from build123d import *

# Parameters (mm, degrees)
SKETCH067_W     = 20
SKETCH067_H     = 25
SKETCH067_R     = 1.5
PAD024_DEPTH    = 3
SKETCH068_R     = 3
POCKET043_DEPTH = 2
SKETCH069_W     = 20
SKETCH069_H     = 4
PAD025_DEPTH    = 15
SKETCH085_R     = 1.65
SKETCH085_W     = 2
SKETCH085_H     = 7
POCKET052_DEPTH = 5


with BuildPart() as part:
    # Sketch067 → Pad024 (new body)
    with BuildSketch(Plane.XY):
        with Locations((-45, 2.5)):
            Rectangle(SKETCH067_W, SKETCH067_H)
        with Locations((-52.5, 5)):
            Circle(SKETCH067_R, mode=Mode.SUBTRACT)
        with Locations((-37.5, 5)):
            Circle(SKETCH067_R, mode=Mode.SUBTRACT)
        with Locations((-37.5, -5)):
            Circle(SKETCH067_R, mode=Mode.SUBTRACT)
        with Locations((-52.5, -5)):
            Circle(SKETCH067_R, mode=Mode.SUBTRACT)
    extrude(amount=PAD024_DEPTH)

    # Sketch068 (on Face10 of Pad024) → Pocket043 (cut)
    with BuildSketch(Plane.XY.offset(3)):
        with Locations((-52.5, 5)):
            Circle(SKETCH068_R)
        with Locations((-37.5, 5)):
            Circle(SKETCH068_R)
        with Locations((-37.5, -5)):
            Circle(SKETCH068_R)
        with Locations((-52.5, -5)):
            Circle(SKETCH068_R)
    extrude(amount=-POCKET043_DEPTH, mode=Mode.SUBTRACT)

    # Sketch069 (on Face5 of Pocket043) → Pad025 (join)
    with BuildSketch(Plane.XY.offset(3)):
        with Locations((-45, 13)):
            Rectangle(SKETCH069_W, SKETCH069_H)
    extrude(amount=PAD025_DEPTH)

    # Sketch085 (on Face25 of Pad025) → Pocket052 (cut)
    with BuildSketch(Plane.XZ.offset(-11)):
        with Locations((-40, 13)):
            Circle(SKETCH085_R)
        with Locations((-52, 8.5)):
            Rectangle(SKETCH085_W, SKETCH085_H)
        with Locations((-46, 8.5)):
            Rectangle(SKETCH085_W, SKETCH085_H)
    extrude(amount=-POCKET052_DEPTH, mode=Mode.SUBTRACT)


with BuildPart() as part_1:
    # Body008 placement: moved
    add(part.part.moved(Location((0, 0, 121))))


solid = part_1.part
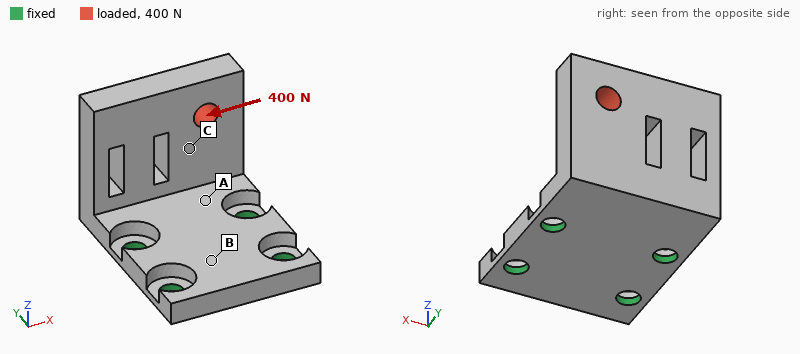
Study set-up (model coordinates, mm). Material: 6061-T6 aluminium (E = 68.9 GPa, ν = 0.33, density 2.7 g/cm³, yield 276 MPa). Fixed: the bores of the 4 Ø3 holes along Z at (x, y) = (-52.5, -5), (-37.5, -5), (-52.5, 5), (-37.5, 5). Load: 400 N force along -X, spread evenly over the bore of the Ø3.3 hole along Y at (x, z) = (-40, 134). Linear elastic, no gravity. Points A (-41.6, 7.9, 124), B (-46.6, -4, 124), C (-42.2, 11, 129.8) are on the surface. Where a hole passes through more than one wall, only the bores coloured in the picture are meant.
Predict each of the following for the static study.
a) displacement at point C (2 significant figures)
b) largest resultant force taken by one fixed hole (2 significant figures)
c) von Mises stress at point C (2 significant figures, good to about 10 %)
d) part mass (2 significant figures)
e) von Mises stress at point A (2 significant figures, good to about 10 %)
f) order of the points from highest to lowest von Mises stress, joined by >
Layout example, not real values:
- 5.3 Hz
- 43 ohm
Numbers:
- 36 µm
- 440 N
- 36 MPa
- 6.2 g
- 68 MPa
- A > C > B
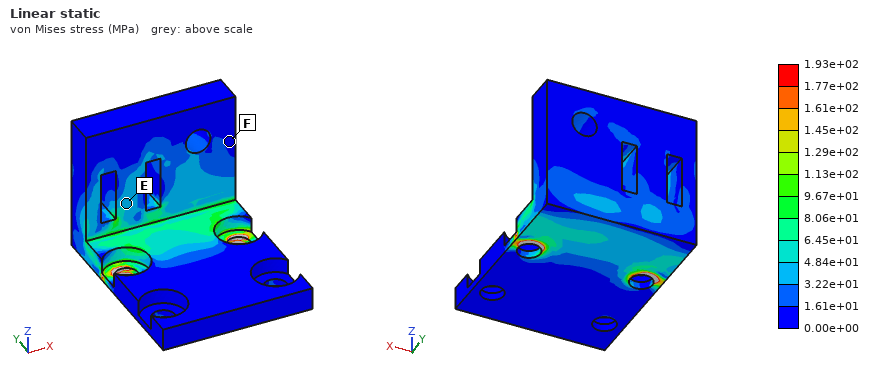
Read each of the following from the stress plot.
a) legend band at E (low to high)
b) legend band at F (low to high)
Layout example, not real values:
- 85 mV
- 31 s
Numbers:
- 3.22e+01 to 4.84e+01 MPa
- 0.00e+00 to 1.61e+01 MPa
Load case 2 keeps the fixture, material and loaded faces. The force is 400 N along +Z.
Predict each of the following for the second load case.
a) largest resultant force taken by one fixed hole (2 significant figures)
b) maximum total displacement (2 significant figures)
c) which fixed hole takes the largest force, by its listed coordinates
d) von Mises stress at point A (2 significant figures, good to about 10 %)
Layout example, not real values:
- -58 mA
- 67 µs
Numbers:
- 530 N
- 0.19 mm
- (-37.5, 5)
- 130 MPa
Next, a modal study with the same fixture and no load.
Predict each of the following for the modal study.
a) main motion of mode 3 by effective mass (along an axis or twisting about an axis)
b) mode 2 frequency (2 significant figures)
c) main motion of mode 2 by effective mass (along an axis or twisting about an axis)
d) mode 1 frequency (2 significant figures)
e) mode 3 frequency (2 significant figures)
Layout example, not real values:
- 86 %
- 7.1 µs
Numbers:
- along Z
- 8100 Hz
- along X
- 3700 Hz
- 14 kHz
